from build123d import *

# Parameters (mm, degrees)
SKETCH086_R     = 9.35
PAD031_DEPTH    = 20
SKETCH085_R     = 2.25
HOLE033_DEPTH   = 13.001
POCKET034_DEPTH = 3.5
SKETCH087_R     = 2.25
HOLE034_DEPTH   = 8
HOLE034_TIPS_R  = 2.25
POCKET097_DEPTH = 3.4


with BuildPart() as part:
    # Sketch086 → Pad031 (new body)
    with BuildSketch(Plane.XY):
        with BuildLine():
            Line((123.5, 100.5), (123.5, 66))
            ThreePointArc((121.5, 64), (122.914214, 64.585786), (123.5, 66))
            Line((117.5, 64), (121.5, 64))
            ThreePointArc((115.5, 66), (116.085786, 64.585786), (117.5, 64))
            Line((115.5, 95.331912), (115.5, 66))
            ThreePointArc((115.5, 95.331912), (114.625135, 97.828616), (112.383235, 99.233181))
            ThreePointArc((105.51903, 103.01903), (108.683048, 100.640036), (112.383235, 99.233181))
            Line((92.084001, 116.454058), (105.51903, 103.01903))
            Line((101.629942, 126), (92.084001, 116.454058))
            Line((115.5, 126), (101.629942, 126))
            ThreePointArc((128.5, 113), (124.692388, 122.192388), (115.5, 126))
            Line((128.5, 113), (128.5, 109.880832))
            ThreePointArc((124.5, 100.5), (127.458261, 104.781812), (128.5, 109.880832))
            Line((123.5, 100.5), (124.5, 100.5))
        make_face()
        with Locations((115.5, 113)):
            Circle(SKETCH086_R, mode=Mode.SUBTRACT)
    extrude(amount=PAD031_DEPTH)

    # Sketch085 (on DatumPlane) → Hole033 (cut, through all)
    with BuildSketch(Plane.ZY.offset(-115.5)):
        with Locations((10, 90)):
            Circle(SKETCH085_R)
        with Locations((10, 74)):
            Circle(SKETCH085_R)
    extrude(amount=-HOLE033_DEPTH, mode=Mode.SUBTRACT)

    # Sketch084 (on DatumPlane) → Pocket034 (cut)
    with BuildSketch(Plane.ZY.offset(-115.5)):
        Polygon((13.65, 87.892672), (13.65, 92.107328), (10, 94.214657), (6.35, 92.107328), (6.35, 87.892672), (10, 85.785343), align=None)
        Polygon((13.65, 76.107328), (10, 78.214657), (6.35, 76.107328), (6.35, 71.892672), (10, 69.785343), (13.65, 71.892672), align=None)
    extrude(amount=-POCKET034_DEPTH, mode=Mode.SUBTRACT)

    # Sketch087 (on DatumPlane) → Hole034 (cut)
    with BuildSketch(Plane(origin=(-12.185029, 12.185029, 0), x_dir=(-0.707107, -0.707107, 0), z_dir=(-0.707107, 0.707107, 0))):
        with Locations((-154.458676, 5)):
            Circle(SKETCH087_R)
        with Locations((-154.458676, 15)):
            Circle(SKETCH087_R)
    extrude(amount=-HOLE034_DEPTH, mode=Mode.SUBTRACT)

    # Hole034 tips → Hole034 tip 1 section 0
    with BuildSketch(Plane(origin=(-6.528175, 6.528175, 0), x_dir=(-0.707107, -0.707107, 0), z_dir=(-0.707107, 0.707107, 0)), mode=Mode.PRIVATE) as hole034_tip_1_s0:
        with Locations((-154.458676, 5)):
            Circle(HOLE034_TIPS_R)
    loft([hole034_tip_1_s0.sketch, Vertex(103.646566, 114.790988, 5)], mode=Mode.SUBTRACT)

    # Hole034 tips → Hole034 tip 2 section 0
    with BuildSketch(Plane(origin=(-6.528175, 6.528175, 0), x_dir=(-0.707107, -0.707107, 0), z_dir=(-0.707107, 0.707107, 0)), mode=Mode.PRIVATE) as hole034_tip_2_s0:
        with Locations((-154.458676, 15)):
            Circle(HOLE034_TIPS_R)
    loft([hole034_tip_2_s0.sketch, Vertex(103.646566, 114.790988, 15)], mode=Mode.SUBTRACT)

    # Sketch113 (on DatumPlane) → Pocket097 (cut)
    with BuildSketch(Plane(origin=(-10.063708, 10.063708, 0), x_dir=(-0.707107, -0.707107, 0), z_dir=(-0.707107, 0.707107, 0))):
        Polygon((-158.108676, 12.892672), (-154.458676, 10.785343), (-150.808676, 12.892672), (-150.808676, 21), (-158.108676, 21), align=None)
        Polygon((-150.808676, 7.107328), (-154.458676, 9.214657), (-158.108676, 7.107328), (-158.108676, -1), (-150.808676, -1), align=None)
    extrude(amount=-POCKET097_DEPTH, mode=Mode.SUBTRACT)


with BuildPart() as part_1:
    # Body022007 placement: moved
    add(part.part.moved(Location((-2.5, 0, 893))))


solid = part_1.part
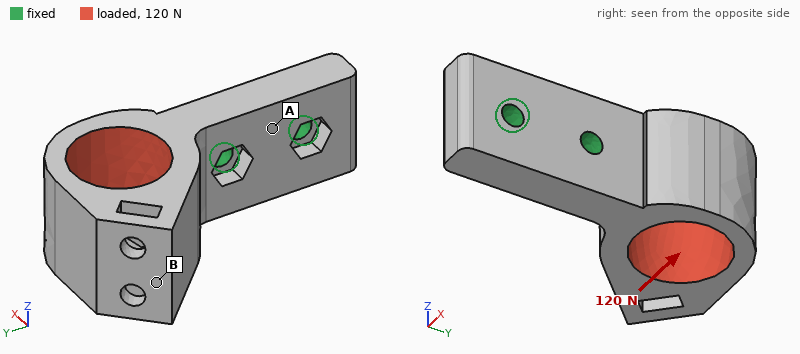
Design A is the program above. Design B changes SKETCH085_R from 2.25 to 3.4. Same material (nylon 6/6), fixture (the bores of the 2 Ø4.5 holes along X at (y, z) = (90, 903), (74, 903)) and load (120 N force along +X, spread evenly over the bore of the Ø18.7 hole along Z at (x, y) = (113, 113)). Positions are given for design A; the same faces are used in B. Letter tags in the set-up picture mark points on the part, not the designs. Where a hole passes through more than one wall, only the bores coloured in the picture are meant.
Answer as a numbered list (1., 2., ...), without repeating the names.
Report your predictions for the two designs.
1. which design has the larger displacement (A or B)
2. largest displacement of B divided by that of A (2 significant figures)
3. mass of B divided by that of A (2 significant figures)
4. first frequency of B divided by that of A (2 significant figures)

1. A
2. 0.83
3. 0.99
4. 1.1
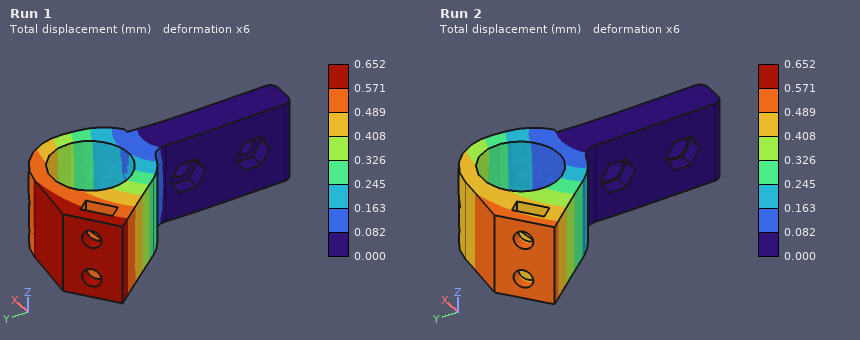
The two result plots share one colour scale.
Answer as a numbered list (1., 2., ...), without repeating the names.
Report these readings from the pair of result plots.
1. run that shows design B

1. Run 2
